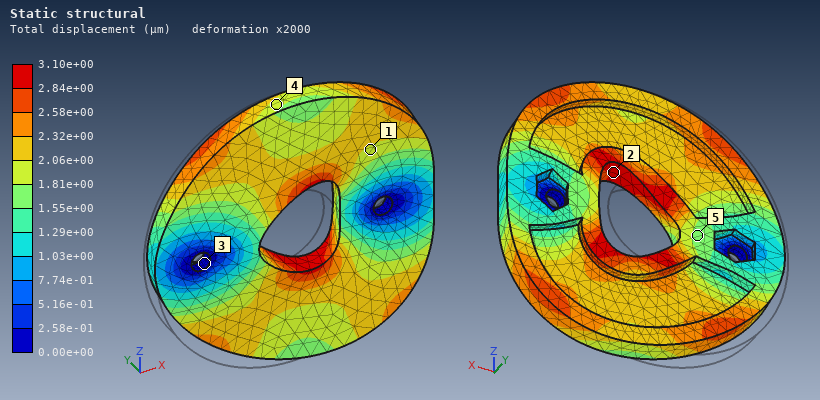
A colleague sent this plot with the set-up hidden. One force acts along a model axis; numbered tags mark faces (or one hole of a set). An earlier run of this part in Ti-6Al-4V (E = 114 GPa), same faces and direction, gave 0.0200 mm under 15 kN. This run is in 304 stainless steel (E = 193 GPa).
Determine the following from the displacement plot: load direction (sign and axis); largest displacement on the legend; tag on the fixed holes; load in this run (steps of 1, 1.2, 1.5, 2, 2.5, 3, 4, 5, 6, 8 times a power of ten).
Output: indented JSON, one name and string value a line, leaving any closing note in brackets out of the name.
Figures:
{
  "load direction": "+X",
  "largest displacement on the legend": "3.10e+00 µm",
  "tag on the fixed holes": "3",
  "load in this run": "4 kN"
}
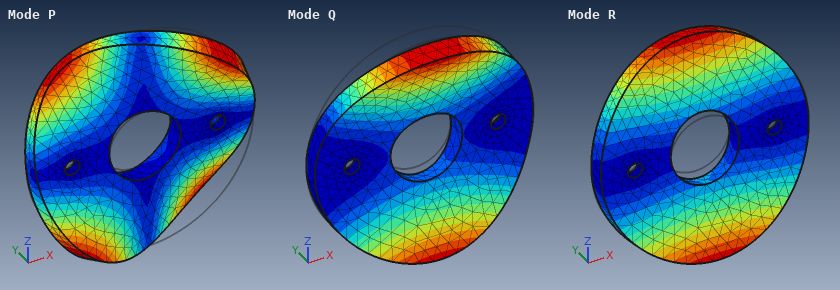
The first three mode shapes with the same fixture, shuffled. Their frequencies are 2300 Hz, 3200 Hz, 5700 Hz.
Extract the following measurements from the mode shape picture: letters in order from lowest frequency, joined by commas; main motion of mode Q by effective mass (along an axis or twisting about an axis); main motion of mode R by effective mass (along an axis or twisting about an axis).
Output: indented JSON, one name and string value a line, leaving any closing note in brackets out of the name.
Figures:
{
  "letters in order from lowest frequency, joined by commas": "R, Q, P",
  "main motion of mode Q by effective mass": "along Y",
  "main motion of mode R by effective mass": "twisting about X"
}
